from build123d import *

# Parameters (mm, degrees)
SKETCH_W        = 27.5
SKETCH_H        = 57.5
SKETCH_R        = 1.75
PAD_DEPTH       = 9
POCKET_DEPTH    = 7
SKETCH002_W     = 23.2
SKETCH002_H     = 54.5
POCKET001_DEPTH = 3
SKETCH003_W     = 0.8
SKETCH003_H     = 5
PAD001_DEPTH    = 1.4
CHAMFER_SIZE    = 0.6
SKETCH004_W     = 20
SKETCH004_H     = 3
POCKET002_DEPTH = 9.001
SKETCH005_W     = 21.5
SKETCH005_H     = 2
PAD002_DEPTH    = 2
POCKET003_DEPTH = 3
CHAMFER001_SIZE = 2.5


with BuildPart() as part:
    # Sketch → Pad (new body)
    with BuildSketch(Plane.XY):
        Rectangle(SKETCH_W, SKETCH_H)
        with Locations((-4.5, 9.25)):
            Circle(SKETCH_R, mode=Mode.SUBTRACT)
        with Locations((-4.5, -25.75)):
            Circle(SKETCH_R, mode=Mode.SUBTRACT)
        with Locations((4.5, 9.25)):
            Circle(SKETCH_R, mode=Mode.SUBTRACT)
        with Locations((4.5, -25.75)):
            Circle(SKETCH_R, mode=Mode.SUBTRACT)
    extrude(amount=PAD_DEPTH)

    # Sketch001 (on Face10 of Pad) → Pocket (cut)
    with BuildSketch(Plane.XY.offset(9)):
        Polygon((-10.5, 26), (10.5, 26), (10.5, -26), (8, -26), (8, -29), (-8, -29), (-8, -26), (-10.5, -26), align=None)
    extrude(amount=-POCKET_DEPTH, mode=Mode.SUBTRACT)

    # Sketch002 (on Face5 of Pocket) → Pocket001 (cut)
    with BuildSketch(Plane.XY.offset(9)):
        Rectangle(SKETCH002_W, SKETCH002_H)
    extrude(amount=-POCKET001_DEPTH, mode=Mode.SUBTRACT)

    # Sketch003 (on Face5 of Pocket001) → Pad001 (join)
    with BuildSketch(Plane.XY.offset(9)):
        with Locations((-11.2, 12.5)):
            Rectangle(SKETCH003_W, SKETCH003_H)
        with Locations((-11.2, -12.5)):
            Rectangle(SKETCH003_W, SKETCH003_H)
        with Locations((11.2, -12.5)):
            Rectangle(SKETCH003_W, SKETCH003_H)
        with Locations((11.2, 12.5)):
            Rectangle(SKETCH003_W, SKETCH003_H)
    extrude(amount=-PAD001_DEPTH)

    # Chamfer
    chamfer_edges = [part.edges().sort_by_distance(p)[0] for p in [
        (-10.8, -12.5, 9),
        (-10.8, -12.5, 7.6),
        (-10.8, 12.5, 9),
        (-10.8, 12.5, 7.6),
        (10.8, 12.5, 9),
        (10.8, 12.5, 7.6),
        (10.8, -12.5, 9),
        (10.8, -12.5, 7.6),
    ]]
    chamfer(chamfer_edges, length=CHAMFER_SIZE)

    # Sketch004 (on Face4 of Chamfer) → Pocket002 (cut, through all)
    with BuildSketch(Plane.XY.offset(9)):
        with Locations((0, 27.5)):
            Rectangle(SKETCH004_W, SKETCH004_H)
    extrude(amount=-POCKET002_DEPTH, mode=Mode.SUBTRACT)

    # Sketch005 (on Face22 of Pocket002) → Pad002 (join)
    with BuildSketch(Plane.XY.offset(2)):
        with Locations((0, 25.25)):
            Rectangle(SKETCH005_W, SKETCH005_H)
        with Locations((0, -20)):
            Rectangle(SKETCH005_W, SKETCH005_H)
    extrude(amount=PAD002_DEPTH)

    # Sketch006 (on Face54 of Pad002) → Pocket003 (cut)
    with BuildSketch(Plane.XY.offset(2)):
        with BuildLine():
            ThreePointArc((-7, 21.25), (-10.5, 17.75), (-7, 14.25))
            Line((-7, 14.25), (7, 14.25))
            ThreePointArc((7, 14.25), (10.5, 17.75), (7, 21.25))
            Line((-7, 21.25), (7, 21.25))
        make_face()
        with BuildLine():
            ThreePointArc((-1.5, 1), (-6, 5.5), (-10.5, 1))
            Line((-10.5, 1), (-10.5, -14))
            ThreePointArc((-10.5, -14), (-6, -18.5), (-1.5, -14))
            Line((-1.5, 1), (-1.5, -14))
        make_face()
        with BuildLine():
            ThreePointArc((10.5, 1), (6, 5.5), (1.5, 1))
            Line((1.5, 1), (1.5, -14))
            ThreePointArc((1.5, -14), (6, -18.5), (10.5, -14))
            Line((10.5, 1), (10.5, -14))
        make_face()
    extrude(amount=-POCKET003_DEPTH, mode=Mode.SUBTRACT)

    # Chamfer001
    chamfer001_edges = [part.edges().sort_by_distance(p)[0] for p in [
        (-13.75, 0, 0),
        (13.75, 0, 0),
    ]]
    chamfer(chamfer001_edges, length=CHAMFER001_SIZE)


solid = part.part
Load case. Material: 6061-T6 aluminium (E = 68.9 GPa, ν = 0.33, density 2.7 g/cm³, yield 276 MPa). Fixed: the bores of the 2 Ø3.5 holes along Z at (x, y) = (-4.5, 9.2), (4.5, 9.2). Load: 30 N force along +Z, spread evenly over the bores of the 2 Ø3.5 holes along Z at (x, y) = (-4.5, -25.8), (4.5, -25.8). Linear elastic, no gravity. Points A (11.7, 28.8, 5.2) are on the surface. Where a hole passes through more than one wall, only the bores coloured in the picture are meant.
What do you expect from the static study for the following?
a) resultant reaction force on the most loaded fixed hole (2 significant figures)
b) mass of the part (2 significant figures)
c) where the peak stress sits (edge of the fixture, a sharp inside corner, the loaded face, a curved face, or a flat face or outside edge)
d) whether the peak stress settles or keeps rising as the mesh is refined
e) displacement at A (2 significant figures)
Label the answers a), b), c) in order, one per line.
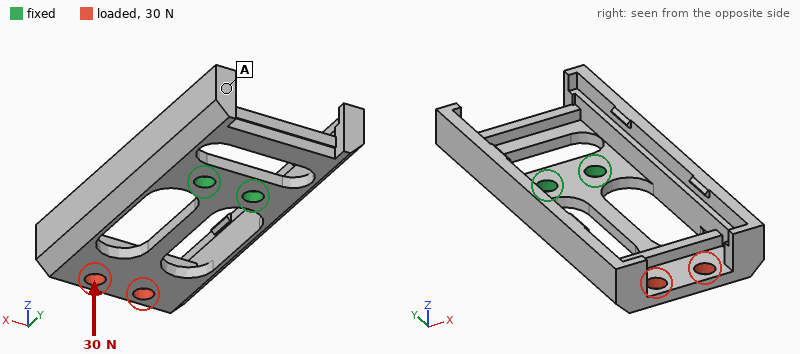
a) 16 N
b) 11 g
c) edge of the fixture
d) keeps rising
e) 0.057 mm
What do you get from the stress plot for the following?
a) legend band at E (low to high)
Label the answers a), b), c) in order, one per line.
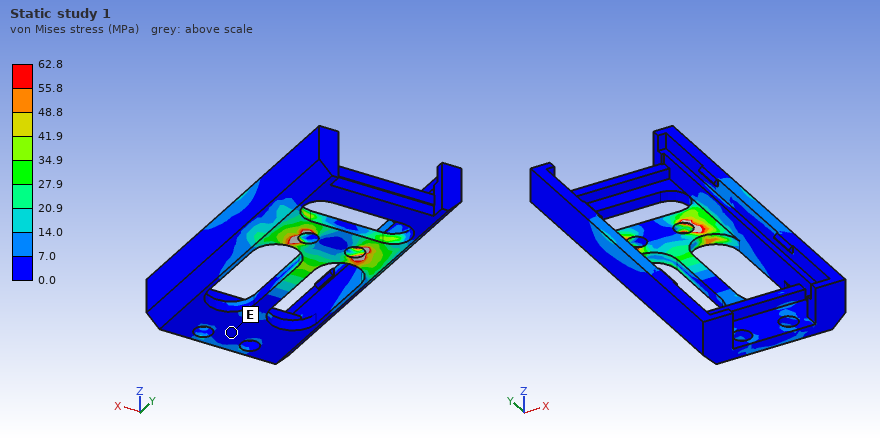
a) 0.0 to 7.0 MPa
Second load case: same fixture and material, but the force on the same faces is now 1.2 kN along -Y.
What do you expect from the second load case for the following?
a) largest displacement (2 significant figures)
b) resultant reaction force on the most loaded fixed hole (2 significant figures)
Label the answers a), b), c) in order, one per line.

a) 85 µm
b) 630 N
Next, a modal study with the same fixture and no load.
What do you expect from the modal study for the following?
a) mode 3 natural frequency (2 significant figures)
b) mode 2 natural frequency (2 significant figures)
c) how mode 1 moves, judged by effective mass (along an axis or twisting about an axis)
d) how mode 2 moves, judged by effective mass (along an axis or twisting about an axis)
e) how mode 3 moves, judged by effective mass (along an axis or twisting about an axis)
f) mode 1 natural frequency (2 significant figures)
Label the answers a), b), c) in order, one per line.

a) 3100 Hz
b) 2300 Hz
c) along Z
d) along X
e) along X
f) 1300 Hz
